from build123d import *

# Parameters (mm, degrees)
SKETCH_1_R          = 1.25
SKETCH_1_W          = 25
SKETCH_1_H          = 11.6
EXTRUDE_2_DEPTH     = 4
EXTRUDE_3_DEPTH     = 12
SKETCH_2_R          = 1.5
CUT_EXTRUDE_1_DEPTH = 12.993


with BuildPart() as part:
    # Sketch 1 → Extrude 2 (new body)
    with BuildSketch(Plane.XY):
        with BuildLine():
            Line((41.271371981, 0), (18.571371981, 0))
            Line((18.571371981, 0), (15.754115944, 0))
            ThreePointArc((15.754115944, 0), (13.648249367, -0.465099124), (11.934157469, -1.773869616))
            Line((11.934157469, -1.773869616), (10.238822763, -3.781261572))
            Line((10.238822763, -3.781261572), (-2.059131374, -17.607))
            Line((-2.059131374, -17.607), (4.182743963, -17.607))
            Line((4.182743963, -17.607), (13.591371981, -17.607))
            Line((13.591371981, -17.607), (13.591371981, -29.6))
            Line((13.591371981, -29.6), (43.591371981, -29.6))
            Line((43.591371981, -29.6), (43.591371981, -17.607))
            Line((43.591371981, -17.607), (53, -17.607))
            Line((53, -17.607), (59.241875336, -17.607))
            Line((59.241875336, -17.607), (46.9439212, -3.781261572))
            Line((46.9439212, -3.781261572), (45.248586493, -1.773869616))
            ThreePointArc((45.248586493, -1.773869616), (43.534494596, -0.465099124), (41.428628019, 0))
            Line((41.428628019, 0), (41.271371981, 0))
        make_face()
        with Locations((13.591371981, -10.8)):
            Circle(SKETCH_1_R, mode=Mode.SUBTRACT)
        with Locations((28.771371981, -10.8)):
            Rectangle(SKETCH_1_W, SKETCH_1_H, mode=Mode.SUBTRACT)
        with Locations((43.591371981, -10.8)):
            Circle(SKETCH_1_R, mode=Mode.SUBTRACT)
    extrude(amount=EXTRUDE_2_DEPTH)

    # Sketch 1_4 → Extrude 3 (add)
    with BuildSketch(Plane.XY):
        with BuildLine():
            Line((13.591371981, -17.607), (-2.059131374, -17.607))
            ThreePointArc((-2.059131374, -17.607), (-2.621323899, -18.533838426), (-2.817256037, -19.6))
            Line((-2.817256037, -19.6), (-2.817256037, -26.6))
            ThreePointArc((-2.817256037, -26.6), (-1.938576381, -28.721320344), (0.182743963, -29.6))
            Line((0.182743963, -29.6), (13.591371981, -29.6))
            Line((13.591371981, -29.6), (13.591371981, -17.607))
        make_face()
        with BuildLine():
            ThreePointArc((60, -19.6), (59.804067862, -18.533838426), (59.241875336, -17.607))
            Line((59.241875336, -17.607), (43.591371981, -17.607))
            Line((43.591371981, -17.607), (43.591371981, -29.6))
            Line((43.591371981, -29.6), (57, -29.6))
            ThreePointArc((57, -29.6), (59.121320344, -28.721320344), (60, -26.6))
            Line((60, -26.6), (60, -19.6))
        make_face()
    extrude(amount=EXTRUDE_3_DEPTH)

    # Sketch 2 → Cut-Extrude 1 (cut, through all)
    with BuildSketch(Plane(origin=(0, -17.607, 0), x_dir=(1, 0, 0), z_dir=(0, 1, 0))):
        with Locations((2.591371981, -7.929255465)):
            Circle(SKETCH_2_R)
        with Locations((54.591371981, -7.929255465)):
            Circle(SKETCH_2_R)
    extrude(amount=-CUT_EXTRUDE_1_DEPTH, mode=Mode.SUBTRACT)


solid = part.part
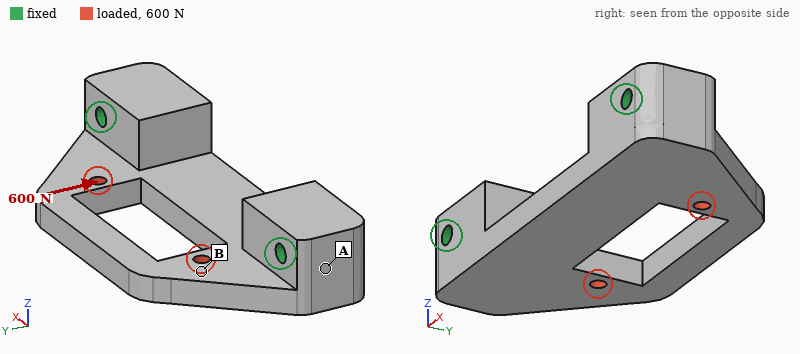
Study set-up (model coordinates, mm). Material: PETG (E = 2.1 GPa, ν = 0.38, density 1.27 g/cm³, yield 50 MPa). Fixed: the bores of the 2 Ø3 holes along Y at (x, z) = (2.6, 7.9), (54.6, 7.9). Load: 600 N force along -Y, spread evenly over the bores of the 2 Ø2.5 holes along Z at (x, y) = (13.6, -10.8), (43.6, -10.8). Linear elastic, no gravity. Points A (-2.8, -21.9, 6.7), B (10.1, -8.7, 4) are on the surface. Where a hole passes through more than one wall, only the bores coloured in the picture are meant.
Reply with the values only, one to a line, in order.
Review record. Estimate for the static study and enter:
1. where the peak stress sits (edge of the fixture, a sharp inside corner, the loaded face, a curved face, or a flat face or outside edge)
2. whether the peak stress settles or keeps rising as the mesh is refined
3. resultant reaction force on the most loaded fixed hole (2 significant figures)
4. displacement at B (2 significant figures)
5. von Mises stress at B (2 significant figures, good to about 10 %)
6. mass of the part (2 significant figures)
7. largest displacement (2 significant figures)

edge of the fixture
keeps rising
310 N
0.11 mm
5.9 MPa
10 g
0.18 mm
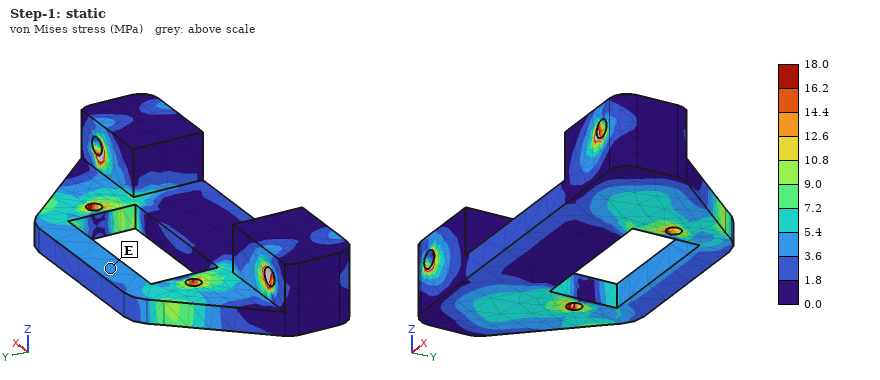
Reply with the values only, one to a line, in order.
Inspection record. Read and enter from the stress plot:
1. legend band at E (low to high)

3.6 to 5.4 MPa
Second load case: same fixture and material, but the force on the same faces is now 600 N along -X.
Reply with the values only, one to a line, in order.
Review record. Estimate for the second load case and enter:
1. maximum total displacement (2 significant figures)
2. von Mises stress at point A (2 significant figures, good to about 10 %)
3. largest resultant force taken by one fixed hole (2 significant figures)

0.23 mm
6.0 MPa
310 N
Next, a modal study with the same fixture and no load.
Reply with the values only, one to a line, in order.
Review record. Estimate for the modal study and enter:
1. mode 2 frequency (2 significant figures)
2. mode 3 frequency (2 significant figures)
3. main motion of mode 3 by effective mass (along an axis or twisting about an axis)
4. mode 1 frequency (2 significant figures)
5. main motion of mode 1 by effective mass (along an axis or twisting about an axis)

3100 Hz
3600 Hz
along Z
1600 Hz
along Z
